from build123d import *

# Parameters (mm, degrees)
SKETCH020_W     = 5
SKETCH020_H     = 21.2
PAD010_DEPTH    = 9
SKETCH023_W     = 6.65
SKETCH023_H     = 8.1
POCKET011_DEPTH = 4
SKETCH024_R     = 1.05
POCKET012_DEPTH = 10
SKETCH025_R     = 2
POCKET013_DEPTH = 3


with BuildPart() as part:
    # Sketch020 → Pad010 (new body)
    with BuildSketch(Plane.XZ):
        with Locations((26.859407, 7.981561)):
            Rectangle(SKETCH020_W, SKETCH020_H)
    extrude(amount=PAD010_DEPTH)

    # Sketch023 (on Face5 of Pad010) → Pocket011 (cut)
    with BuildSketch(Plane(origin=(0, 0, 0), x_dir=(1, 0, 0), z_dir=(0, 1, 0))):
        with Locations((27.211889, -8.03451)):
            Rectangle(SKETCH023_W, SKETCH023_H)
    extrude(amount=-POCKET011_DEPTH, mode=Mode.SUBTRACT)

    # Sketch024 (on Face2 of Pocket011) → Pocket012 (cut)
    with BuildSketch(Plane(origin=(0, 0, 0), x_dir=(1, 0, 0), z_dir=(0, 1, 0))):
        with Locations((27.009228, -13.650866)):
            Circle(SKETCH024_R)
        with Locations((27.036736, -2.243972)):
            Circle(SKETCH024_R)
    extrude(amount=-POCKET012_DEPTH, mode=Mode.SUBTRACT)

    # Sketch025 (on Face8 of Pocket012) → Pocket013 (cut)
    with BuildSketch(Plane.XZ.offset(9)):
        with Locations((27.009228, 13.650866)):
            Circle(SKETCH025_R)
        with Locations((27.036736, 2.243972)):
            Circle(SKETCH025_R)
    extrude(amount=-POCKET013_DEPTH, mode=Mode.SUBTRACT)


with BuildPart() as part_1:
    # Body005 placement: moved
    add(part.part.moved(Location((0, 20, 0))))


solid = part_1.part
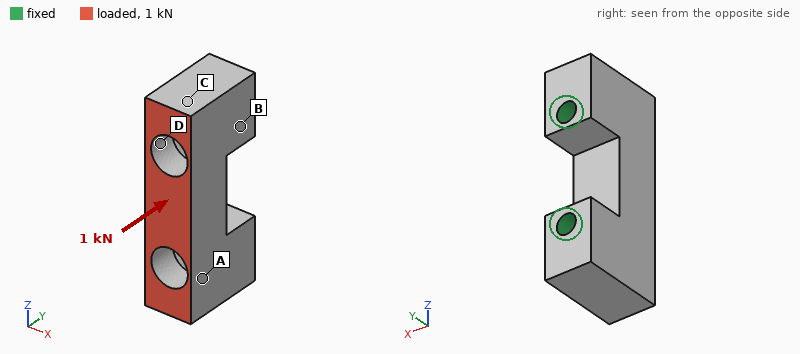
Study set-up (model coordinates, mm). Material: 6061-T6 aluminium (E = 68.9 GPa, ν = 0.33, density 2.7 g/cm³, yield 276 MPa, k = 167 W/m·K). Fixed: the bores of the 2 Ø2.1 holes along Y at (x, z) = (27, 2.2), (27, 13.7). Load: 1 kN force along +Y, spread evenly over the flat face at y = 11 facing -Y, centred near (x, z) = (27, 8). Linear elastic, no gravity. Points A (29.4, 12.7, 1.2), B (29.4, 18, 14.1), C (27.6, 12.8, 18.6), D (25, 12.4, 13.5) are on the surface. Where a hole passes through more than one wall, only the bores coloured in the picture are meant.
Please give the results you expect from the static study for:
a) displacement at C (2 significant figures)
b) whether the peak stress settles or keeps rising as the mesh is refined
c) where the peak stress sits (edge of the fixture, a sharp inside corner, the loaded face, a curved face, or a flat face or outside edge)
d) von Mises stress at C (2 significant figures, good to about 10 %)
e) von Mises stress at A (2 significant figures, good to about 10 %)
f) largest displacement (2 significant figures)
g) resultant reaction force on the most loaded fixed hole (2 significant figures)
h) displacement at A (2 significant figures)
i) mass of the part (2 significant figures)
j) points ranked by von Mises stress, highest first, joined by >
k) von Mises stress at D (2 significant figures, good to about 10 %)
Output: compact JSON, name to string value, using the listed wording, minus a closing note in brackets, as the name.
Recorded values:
{"displacement at C": "1.8 µm", "whether the peak stress settles or keeps rising as the mesh is refined": "keeps rising", "where the peak stress sits": "edge of the fixture", "von Mises stress at C": "11 MPa", "von Mises stress at A": "19 MPa", "largest displacement": "3.2 µm", "resultant reaction force on the most loaded fixed hole": "510 N", "displacement at A": "1.0 µm", "mass of the part": "1.8 g", "points ranked by von Mises stress, highest first, joined by >": "D > A > C > B", "von Mises stress at D": "24 MPa"}
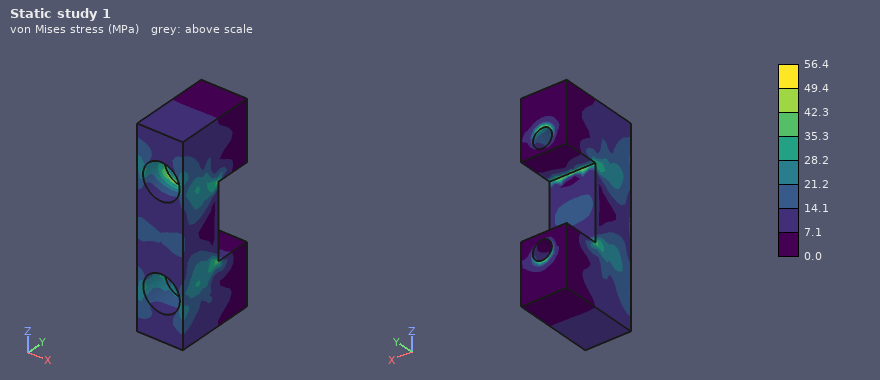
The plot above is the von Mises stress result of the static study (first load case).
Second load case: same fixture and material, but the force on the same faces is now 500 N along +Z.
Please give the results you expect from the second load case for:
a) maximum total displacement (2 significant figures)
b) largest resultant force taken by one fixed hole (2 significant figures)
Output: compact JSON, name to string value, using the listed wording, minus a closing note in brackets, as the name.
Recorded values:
{"maximum total displacement": "4.0 µm", "largest resultant force taken by one fixed hole": "280 N"}
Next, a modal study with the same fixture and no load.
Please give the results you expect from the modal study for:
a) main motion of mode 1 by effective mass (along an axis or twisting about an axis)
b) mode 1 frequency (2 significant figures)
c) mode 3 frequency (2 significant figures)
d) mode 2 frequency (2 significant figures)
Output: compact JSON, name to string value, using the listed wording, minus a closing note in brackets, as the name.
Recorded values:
{"main motion of mode 1 by effective mass": "along X", "mode 1 frequency": "63 kHz", "mode 3 frequency": "75 kHz", "mode 2 frequency": "73 kHz"}
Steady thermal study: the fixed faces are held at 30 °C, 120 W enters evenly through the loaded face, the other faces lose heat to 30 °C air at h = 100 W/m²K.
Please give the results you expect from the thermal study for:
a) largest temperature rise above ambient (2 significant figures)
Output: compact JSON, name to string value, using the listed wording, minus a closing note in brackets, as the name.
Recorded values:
{"largest temperature rise above ambient": "66 K"}
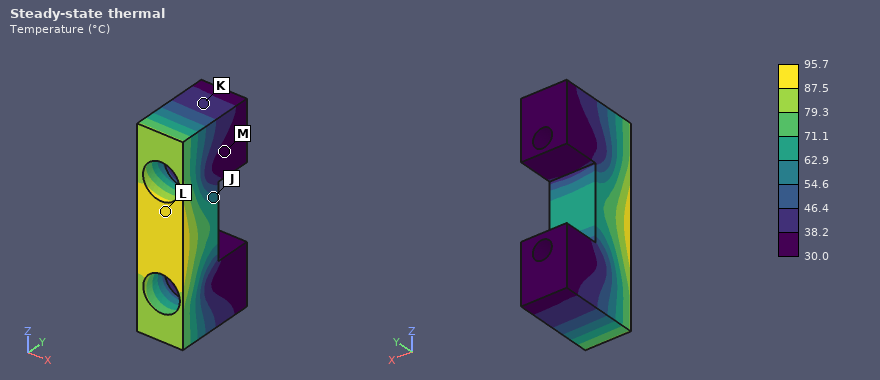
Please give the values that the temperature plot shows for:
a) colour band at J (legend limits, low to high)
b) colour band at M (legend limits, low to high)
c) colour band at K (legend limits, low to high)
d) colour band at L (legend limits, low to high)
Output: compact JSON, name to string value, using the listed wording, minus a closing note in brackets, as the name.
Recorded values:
{"colour band at J": "54.6 to 62.9 °C", "colour band at M": "30.0 to 38.2 °C", "colour band at K": "38.2 to 46.4 °C", "colour band at L": "87.5 to 95.7 °C"}
